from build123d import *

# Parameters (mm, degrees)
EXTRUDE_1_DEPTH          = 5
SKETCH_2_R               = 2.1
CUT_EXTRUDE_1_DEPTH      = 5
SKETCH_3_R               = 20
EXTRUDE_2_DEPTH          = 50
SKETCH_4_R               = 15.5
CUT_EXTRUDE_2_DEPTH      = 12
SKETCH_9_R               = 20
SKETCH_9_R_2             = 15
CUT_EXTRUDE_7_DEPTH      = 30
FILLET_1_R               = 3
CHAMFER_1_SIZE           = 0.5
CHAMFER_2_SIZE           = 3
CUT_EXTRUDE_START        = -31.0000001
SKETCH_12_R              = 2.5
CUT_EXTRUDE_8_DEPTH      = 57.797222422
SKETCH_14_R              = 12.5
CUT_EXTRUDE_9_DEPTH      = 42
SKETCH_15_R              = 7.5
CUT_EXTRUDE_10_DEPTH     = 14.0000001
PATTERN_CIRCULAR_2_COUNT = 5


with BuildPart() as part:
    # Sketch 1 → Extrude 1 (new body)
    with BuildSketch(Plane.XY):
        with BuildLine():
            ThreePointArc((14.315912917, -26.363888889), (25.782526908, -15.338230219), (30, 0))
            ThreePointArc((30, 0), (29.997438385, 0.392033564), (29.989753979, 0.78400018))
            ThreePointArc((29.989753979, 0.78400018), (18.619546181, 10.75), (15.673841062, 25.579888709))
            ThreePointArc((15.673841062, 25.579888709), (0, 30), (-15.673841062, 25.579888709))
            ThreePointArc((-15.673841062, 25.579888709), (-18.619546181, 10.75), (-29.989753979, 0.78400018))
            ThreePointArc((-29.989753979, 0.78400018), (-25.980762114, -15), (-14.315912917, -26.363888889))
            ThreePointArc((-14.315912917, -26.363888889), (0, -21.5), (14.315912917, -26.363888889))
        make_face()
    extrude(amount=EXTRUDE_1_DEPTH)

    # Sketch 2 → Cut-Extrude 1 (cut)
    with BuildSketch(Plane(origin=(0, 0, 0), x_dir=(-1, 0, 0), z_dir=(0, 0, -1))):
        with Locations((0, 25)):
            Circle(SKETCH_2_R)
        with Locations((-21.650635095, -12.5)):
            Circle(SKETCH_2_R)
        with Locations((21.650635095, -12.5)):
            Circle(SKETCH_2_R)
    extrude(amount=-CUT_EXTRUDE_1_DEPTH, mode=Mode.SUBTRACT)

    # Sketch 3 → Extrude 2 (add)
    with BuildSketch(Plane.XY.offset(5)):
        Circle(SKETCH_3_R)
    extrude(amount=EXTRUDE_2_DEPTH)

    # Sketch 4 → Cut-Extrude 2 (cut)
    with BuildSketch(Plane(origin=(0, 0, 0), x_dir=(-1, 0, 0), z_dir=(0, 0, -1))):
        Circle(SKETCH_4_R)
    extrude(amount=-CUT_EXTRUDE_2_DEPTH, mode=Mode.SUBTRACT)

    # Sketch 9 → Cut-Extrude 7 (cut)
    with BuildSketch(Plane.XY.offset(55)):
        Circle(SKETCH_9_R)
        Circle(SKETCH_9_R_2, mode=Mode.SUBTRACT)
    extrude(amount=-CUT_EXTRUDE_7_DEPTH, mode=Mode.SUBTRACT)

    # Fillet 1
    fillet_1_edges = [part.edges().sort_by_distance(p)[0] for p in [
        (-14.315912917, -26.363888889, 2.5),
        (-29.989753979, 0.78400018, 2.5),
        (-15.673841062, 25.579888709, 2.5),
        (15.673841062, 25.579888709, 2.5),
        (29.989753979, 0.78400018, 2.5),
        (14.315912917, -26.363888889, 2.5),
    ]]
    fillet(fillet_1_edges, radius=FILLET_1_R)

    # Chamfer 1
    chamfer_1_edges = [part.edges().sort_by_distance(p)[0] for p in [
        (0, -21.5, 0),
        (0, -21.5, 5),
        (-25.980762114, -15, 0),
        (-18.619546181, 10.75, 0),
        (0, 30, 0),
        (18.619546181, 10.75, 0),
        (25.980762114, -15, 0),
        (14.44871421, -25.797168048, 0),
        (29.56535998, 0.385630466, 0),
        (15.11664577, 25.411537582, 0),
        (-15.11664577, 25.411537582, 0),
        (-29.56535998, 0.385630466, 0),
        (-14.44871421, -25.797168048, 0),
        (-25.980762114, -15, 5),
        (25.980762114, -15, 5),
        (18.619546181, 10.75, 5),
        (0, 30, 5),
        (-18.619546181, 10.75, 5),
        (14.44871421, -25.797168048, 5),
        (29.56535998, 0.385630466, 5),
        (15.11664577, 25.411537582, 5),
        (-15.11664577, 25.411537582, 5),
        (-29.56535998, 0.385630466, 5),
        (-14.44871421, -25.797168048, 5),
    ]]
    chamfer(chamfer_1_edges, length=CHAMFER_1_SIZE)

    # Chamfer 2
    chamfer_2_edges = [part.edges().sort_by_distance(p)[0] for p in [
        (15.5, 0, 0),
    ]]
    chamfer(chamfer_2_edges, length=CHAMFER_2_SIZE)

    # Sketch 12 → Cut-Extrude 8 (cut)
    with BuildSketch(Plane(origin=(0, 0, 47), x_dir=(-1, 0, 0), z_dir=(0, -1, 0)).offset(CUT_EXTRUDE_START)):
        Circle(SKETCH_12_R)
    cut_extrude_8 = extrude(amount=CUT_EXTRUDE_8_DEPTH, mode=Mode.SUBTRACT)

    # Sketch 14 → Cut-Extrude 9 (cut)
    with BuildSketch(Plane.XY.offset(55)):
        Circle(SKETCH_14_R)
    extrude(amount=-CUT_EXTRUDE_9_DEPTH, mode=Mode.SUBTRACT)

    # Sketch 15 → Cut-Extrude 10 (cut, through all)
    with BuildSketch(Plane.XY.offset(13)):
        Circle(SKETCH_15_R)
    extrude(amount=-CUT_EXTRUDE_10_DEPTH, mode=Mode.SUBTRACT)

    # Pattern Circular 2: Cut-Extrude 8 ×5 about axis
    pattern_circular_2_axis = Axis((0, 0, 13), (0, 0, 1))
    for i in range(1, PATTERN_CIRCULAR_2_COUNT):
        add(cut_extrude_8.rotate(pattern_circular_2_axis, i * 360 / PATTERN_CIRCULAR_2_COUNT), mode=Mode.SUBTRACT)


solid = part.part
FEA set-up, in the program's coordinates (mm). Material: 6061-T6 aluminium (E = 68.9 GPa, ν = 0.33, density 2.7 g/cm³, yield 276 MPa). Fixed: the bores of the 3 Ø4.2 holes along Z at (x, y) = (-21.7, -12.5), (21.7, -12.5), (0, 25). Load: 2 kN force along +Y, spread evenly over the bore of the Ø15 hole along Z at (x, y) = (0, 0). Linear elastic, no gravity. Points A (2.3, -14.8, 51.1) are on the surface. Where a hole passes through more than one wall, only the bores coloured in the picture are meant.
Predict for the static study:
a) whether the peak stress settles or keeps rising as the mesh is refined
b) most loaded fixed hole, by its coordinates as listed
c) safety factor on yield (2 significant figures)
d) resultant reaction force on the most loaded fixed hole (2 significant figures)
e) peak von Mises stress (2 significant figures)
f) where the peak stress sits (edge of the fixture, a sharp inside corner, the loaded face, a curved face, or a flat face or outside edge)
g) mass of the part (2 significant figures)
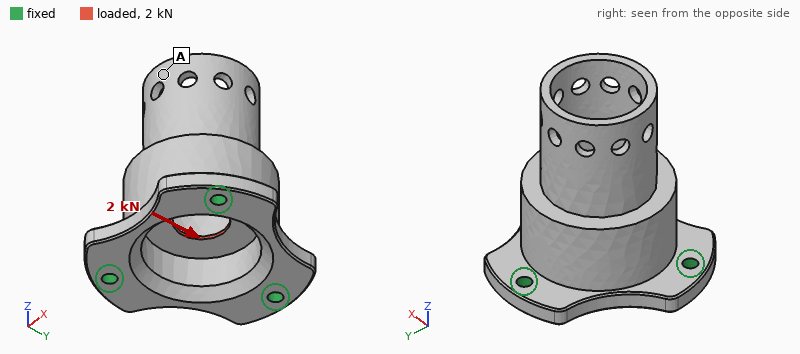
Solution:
settles
(0, 25)
3.6
840 N
77 MPa
the loaded face
73 g
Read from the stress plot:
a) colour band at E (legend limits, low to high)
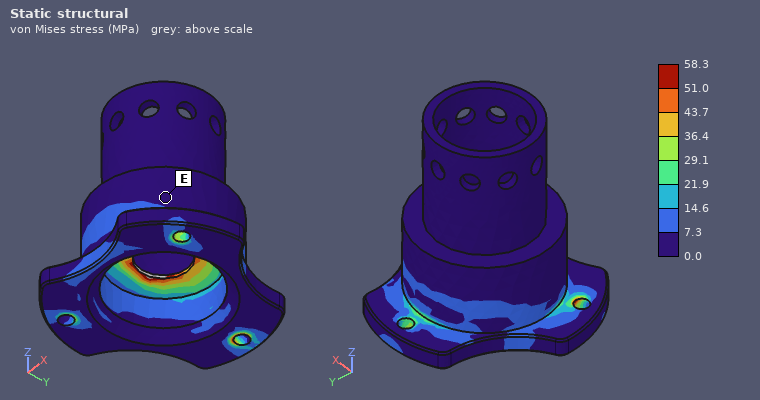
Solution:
0.0 to 7.3 MPa
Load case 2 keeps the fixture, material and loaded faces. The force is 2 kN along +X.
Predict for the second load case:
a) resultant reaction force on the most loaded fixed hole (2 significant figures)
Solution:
810 N
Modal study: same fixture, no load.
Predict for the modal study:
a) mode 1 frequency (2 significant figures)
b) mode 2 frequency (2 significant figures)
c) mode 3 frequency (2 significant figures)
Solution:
6300 Hz
6400 Hz
11 kHz
